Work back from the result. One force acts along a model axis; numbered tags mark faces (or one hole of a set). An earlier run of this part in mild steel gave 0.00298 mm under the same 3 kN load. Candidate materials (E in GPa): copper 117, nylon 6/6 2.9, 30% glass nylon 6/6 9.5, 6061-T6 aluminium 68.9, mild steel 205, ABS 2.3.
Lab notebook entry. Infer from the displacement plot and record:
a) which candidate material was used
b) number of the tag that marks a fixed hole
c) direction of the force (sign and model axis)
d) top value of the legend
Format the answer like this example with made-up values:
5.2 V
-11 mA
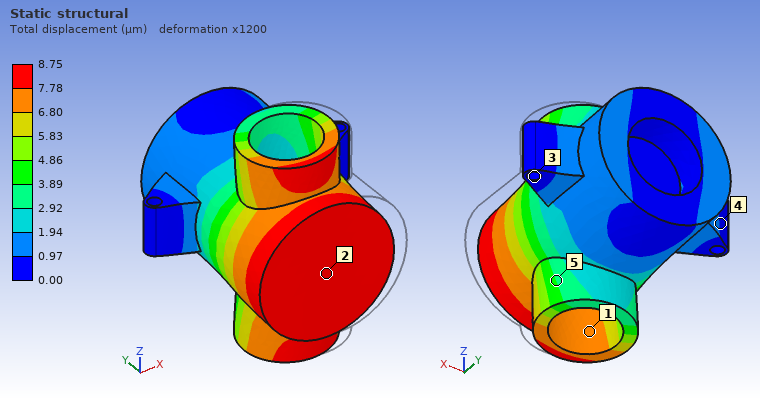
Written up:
6061-T6 aluminium
3
-X
8.75 µm
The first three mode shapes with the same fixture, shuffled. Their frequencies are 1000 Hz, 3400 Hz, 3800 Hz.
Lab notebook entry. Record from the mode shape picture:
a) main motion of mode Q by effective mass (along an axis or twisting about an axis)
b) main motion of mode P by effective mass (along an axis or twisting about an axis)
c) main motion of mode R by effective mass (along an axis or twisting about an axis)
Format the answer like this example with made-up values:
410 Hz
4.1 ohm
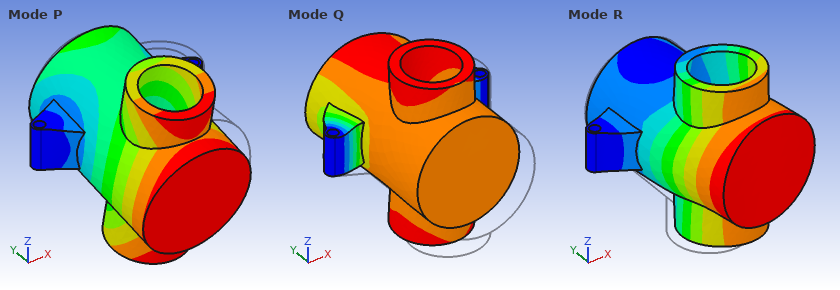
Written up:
along Y
along Z
along X
